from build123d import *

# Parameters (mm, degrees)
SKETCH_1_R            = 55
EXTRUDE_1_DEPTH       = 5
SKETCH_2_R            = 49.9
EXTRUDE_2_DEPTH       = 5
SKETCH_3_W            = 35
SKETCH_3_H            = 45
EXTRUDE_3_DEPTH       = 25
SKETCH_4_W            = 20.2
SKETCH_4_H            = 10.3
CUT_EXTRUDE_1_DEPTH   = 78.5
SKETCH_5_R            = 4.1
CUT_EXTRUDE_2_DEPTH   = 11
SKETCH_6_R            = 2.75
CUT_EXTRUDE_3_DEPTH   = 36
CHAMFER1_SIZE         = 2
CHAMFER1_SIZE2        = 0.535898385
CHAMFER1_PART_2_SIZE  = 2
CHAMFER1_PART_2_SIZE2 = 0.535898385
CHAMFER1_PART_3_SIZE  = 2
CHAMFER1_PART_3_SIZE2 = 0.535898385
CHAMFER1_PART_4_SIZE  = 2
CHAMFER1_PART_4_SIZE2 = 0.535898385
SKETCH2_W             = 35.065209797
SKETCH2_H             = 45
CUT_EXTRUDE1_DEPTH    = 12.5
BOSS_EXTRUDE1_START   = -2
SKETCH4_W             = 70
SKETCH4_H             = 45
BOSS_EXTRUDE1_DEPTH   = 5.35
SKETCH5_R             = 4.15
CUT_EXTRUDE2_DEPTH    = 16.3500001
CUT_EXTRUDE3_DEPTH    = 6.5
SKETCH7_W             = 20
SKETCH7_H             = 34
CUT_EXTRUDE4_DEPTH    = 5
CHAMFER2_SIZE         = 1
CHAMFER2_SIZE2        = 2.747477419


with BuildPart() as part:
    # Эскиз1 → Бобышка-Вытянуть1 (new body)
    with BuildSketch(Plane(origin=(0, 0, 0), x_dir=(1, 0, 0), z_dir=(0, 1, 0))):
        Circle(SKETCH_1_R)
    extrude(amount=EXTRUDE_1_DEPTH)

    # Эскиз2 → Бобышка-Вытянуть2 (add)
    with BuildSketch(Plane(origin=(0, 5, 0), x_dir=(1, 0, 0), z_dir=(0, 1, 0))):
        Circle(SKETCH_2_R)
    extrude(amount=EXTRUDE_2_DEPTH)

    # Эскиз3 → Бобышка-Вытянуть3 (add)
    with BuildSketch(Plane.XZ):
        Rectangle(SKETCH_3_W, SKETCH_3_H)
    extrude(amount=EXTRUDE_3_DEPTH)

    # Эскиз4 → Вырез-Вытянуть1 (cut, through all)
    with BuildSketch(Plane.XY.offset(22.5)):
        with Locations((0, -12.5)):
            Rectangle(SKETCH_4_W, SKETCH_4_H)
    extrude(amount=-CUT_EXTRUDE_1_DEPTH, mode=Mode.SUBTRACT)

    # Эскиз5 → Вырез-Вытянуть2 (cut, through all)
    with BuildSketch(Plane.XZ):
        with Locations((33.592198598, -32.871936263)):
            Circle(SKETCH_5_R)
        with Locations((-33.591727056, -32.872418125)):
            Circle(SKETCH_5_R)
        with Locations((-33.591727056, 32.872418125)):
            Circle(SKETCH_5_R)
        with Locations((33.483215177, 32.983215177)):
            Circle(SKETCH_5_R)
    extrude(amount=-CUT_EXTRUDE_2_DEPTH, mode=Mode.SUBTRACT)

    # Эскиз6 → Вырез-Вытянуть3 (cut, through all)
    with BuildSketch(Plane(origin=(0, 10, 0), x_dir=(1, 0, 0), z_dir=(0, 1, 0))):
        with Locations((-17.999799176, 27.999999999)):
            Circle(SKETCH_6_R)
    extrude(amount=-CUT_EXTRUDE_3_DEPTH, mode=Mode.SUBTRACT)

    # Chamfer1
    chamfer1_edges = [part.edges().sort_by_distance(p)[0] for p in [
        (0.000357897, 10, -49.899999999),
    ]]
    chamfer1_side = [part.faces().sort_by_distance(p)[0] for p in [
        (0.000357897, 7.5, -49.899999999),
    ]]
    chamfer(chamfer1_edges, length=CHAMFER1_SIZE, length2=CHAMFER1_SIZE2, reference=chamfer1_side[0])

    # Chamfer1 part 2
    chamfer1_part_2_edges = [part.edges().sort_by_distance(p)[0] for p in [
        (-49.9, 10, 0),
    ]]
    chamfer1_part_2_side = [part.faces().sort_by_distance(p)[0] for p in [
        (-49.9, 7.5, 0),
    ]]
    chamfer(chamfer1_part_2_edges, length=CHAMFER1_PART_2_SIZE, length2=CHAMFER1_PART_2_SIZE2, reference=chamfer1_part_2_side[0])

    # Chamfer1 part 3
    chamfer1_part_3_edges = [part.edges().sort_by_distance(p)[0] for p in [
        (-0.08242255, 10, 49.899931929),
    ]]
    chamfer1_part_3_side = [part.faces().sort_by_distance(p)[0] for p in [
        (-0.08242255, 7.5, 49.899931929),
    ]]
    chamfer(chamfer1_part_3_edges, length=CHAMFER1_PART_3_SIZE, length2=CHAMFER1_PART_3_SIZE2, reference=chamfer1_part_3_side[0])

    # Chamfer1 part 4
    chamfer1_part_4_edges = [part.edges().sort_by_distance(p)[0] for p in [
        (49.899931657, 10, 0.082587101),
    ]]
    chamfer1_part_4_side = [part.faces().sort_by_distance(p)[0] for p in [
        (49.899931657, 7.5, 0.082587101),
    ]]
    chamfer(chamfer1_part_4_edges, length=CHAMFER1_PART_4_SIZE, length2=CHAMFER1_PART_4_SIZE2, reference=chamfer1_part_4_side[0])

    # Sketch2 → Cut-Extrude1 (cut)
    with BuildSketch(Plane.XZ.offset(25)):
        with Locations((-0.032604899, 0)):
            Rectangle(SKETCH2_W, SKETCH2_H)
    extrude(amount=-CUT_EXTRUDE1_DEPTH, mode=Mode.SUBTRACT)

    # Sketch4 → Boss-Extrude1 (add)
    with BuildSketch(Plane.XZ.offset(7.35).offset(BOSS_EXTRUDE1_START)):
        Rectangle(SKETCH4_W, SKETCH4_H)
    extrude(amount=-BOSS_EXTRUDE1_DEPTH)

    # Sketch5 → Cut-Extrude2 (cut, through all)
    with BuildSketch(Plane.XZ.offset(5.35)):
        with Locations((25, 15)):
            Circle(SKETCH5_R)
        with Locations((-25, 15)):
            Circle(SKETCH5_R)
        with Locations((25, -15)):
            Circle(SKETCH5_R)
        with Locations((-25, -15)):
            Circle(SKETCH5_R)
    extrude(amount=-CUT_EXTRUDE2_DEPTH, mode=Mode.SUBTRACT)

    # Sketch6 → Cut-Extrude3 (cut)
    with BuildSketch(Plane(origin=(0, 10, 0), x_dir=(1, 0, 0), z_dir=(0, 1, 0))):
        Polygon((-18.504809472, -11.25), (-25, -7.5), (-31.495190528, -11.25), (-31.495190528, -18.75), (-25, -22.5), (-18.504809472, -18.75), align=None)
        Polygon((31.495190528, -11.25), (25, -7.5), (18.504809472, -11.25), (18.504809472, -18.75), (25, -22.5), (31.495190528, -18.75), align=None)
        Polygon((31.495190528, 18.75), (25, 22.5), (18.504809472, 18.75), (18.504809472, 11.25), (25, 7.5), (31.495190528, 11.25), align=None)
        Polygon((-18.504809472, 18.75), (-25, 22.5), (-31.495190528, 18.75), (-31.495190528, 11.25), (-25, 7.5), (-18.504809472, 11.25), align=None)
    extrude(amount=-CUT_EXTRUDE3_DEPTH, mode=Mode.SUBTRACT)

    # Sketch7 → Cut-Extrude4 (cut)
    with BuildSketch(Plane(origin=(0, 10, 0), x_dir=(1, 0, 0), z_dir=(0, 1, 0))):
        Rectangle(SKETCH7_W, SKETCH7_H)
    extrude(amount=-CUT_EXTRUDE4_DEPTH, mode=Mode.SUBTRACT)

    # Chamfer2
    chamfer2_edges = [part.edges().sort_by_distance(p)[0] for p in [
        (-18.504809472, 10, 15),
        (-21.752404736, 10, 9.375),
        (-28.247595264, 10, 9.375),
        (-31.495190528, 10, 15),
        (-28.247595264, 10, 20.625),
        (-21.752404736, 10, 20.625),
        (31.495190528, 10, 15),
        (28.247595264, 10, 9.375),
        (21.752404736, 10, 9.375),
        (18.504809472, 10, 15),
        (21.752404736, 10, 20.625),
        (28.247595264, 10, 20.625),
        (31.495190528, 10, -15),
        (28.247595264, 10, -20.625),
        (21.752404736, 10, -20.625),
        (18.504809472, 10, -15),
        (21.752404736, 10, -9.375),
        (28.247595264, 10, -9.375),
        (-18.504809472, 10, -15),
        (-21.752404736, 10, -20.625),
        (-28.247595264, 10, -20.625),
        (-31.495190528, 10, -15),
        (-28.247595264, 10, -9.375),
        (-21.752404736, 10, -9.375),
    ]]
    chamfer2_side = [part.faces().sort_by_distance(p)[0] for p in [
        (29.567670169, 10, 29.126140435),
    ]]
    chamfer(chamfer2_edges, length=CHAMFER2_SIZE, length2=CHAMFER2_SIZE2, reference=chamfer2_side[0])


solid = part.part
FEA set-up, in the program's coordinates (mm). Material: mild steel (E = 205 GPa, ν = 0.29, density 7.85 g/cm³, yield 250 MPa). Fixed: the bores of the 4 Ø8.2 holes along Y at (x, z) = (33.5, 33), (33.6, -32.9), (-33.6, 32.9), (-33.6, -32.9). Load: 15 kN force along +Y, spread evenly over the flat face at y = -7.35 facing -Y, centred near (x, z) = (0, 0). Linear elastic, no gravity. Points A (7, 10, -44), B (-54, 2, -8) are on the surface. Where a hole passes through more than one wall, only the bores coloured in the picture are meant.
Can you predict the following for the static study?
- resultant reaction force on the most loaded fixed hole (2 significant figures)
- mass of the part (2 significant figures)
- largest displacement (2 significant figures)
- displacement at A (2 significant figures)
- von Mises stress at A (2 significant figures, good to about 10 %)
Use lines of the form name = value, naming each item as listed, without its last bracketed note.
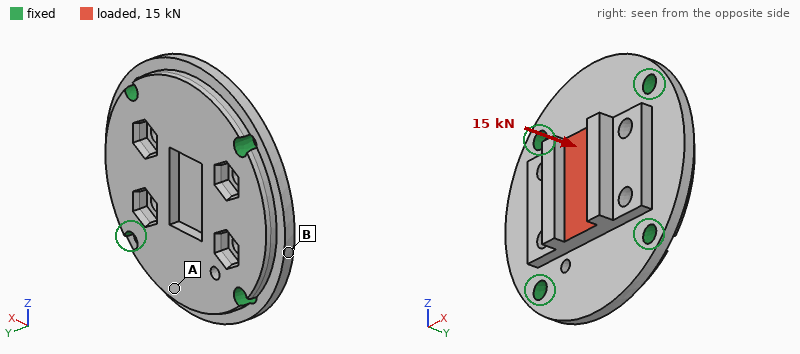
resultant reaction force on the most loaded fixed hole = 4.6 kN
mass of the part = 770 g
largest displacement = 22 µm
displacement at A = 6.4 µm
von Mises stress at A = 27 MPa
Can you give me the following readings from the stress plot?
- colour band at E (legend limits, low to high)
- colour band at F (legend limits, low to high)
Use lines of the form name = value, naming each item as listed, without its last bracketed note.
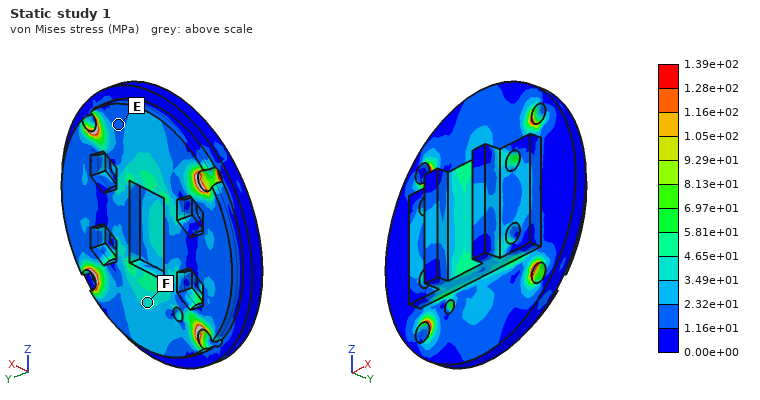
colour band at E = 1.16e+01 to 2.32e+01 MPa
colour band at F = 3.49e+01 to 4.65e+01 MPa
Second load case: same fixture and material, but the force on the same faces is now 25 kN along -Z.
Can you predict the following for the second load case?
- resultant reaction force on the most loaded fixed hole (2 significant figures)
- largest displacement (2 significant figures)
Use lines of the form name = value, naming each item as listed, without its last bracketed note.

resultant reaction force on the most loaded fixed hole = 7.2 kN
largest displacement = 16 µm
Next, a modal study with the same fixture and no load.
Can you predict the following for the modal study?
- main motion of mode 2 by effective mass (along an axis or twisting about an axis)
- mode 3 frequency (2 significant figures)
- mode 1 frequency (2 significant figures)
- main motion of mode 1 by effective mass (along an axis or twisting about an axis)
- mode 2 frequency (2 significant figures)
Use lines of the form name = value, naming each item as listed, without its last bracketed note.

main motion of mode 2 by effective mass = twisting about X
mode 3 frequency = 10 kHz
mode 1 frequency = 8100 Hz
main motion of mode 1 by effective mass = along Y
mode 2 frequency = 9700 Hz
